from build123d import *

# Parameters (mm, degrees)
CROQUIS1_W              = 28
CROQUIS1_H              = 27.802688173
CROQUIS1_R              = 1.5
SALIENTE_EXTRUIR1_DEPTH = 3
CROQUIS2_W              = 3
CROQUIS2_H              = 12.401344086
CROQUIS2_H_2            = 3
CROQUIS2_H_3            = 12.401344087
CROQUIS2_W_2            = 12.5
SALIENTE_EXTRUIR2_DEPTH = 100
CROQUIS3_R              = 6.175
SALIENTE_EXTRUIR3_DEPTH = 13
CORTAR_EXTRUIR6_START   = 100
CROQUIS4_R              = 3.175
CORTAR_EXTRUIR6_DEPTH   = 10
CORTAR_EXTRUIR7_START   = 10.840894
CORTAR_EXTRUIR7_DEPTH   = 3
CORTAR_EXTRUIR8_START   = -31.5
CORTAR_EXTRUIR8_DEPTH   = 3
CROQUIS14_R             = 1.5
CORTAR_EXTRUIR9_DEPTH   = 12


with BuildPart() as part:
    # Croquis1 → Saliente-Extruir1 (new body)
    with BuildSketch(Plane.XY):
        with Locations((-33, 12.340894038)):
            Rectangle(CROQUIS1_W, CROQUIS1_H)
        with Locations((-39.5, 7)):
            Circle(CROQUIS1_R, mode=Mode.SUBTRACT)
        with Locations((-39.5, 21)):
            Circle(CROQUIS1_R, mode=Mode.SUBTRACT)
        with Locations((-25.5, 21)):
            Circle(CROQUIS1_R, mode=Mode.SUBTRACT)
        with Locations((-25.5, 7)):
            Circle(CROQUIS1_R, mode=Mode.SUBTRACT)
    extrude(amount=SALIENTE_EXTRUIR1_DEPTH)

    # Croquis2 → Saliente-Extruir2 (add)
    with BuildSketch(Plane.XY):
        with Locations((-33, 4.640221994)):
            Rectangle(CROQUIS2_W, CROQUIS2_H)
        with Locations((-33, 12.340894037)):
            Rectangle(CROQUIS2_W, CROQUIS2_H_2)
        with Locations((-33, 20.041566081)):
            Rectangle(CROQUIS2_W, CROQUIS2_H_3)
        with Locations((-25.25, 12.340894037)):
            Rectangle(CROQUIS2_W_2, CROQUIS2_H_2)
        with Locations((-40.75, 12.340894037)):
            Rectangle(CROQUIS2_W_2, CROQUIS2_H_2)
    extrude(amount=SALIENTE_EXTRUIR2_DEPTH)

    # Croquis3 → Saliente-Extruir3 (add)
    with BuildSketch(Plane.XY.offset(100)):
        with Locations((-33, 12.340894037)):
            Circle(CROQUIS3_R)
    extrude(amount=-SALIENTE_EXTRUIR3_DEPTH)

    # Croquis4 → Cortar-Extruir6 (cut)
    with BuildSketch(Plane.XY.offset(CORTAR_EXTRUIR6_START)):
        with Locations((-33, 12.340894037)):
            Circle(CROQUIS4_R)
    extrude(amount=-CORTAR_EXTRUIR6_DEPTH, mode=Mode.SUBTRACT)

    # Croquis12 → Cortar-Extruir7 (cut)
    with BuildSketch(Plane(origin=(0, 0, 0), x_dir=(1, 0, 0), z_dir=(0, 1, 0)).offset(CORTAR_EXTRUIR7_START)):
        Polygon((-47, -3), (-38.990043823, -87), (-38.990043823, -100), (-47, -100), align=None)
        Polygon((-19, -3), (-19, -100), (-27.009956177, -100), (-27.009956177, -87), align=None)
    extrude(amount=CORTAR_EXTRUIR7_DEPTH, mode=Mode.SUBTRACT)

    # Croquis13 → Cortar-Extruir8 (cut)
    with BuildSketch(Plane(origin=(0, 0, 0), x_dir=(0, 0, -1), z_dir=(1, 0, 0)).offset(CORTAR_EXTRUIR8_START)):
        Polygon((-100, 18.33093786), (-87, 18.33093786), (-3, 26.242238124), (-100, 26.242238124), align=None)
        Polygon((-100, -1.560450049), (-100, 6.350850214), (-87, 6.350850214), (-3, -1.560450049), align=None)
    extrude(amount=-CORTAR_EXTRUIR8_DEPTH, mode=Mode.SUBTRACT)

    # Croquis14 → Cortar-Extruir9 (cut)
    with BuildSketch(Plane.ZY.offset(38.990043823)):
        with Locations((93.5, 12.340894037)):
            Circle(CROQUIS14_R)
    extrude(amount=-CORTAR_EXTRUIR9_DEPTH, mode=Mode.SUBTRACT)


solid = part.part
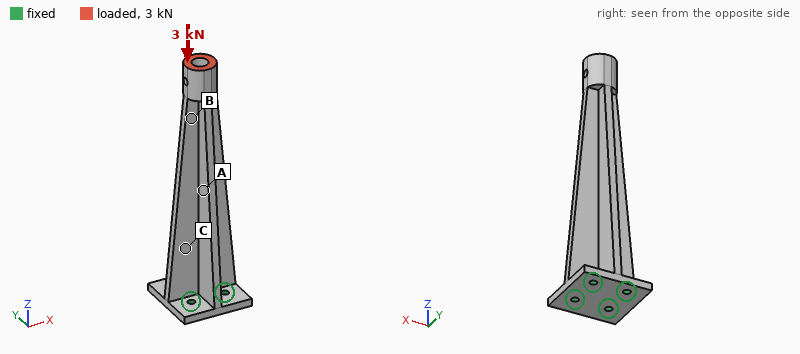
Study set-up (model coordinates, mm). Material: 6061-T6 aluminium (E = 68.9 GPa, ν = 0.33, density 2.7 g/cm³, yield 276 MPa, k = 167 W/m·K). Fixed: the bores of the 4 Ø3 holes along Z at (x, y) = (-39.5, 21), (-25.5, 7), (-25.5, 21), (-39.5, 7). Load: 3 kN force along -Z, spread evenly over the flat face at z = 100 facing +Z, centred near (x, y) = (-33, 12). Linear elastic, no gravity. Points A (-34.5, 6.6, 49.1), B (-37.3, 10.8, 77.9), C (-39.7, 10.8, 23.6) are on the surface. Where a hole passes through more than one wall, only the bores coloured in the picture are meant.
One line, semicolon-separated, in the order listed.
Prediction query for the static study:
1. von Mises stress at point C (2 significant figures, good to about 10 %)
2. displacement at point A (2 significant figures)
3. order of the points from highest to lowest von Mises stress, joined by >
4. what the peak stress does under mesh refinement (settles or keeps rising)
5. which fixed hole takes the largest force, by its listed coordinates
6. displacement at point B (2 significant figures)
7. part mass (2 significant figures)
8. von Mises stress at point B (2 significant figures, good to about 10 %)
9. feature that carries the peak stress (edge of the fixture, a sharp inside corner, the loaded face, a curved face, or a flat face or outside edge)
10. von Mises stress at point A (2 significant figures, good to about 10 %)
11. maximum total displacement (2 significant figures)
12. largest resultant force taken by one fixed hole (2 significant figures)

22 MPa; 24 µm; B > A > C; keeps rising; (-39.5, 7); 38 µm; 34 g; 41 MPa; edge of the fixture; 28 MPa; 53 µm; 1.0 kN
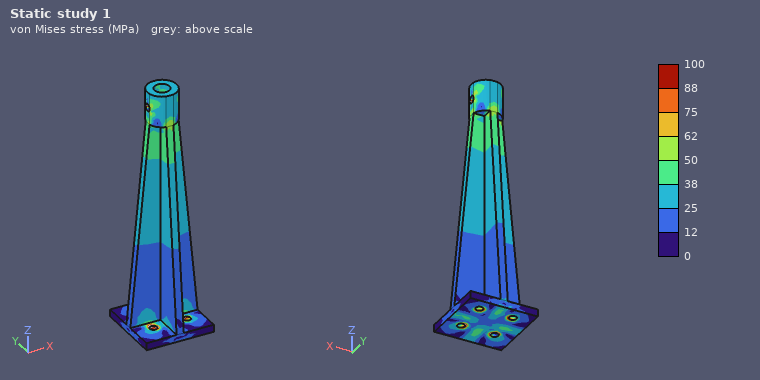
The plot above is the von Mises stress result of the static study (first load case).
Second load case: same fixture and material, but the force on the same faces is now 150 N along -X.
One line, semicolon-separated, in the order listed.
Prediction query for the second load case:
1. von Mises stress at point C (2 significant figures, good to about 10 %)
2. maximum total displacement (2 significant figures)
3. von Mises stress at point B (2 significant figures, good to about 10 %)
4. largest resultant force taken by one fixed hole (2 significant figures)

22 MPa; 0.34 mm; 22 MPa; 610 N
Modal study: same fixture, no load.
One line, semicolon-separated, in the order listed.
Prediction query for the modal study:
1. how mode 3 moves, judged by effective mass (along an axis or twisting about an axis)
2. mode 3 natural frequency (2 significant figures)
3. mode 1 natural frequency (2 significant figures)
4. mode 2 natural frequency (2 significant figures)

twisting about Z; 3500 Hz; 1400 Hz; 1500 Hz
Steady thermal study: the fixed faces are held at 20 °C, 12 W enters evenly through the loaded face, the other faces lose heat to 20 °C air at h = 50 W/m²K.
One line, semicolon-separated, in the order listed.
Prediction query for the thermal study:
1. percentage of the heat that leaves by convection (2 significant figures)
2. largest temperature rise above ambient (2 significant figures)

52 %; 50 K
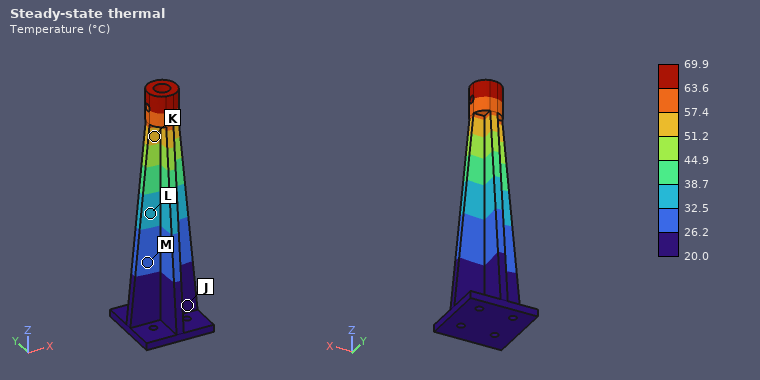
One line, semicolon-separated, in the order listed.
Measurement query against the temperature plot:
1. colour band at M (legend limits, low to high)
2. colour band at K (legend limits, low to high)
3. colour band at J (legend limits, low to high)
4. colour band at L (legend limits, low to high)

26.2 to 32.5 °C; 51.2 to 57.4 °C; 20.0 to 26.2 °C; 32.5 to 38.7 °C
